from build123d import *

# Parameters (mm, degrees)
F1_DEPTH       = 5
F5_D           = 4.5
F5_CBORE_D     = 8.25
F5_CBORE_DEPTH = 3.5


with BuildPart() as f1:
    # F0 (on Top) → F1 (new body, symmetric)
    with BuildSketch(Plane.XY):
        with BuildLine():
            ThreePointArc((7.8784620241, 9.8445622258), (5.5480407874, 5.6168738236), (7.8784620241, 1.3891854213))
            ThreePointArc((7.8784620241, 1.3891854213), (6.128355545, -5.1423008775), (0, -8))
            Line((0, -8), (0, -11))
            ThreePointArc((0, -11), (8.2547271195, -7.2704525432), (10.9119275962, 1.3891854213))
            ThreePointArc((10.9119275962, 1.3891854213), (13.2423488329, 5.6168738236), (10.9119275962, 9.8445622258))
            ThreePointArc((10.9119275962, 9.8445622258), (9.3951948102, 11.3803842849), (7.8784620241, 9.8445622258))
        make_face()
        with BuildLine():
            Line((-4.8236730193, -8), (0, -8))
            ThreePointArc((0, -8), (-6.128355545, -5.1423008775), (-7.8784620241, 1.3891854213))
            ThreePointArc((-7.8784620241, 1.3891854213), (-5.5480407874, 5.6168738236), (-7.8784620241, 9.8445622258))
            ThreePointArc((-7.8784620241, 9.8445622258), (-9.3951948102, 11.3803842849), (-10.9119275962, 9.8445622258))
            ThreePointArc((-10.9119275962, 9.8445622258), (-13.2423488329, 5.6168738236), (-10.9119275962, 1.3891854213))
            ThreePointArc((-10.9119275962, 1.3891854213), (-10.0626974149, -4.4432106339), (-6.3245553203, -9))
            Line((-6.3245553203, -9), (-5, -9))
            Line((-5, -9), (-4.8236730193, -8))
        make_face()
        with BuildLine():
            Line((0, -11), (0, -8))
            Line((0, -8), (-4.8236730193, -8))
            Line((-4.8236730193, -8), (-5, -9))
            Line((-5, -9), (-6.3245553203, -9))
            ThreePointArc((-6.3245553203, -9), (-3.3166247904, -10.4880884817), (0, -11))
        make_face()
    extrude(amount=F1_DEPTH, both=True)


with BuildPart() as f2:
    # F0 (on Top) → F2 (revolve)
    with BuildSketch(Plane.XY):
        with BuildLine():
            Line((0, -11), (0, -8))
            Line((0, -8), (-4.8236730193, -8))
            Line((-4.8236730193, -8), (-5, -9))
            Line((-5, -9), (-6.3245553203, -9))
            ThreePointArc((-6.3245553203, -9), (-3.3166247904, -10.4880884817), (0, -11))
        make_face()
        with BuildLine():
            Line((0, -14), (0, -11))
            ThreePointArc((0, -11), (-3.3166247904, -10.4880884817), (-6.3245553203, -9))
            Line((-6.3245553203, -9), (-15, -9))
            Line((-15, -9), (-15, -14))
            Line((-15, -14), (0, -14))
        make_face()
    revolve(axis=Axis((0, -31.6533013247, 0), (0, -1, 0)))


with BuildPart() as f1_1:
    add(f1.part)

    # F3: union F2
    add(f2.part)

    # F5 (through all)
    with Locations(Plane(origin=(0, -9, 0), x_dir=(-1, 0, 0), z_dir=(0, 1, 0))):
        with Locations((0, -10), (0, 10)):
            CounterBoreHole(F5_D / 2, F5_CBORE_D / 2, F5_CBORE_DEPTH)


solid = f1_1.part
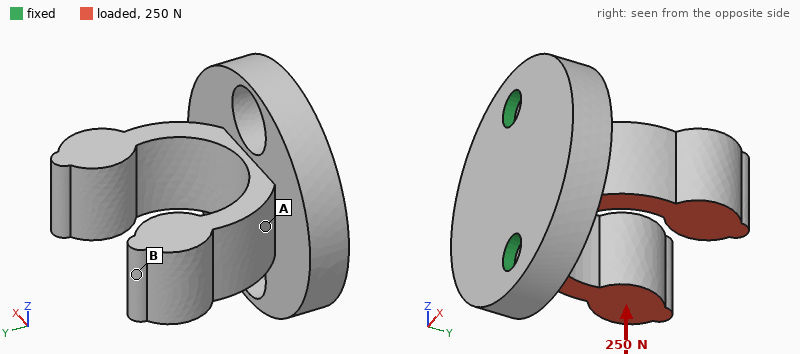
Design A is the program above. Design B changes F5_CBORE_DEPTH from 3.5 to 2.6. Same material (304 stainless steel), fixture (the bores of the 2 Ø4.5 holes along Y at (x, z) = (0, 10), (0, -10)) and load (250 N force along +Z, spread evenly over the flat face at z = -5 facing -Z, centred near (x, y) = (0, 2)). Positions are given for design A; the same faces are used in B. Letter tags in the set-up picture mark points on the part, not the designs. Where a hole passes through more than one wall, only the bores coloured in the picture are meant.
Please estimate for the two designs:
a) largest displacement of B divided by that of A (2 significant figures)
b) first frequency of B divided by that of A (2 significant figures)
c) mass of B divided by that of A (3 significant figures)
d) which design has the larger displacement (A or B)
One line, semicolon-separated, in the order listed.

0.92; 1.2; 1.01; A
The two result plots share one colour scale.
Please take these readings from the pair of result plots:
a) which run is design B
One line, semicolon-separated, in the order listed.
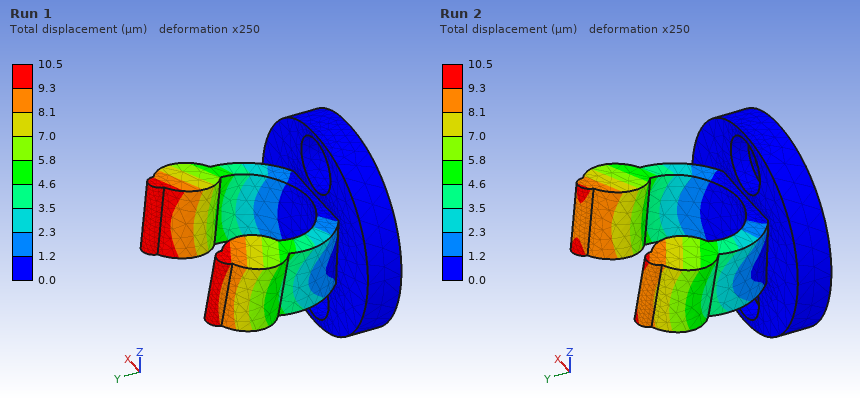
Run 2
